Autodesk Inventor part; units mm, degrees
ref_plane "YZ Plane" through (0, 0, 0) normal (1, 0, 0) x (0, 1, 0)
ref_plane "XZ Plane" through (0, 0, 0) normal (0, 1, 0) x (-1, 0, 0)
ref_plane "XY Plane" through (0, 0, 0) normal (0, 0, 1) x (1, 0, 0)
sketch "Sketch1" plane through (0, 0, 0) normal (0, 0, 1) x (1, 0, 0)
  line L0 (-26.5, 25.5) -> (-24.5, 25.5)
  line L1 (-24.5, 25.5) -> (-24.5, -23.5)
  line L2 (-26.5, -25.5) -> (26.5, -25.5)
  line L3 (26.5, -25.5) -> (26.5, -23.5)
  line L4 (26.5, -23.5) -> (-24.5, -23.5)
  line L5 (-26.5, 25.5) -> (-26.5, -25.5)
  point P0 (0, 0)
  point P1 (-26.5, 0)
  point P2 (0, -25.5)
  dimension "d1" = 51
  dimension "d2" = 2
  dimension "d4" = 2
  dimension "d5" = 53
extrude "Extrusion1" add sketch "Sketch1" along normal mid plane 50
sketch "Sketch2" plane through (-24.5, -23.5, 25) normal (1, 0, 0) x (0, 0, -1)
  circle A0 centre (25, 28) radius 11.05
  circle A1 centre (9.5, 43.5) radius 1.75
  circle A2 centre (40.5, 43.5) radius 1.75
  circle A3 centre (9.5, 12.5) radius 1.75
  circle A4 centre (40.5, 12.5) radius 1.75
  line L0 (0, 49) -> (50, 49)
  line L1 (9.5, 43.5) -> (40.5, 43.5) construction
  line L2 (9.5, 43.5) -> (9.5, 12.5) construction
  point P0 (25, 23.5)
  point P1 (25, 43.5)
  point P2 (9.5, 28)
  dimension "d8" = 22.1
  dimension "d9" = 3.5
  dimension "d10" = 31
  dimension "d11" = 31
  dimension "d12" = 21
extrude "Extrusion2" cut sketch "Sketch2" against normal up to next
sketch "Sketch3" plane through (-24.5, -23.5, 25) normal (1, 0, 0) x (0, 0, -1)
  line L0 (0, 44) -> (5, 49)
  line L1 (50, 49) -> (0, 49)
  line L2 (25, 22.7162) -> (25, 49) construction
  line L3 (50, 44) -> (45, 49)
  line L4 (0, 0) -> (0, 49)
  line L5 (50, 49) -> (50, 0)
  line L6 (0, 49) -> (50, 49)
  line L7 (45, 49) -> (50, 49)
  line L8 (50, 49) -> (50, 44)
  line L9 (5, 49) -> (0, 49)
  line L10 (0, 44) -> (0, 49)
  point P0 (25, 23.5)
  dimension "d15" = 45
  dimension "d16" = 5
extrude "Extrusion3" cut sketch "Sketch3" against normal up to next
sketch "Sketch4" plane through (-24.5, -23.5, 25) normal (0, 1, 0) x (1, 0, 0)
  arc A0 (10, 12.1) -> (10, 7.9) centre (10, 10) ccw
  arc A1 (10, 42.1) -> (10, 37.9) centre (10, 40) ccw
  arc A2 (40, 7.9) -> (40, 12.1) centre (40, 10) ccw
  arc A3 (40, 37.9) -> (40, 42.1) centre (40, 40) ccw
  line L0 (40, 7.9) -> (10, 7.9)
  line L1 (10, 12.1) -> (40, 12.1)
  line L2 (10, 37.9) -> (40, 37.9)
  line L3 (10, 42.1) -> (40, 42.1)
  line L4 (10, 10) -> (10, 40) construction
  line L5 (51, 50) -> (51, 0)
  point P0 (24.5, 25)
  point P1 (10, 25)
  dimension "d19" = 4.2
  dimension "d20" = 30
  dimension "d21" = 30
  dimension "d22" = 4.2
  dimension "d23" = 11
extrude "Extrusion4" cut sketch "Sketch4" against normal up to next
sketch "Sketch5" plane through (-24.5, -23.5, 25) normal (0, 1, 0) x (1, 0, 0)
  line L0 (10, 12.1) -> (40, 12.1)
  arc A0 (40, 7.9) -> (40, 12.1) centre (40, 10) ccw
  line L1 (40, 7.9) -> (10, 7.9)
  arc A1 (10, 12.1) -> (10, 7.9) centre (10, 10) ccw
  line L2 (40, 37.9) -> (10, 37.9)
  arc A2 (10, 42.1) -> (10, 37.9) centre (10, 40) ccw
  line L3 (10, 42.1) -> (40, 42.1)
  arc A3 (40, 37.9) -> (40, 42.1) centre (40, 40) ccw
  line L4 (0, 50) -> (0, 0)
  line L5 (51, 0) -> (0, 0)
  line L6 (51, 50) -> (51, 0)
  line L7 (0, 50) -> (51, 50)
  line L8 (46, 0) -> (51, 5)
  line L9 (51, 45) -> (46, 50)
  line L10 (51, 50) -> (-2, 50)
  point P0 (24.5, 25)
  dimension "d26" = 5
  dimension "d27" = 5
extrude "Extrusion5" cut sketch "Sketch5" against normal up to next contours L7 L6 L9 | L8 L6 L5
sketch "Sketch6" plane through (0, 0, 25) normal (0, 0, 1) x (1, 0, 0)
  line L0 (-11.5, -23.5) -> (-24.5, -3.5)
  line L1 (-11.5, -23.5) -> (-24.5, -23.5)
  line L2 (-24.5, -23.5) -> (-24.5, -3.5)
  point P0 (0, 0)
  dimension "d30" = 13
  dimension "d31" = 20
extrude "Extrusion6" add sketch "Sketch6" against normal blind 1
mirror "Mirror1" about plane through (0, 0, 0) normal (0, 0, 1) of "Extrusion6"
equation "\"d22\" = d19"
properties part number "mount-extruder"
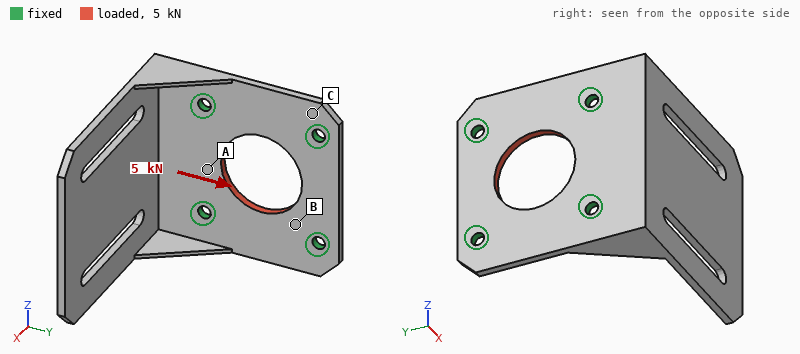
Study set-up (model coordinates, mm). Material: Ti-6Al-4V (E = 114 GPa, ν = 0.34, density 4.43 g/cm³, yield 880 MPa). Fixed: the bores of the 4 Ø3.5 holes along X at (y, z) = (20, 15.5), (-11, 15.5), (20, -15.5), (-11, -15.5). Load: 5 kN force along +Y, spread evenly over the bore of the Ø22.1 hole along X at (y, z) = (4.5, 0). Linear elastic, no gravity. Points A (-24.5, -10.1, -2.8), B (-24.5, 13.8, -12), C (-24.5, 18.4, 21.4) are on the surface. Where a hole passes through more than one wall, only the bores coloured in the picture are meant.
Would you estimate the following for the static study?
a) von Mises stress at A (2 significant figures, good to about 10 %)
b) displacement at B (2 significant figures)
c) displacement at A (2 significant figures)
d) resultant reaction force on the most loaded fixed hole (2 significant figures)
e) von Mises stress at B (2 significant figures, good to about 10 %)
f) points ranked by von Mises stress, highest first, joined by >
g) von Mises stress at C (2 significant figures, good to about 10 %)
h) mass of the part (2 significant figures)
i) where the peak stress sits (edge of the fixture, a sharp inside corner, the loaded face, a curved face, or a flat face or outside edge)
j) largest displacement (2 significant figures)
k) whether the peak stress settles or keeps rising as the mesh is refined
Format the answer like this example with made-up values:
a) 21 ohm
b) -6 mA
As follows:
a) 29 MPa
b) 4.6 µm
c) 6.7 µm
d) 1.3 kN
e) 53 MPa
f) B > A > C
g) 12 MPa
h) 40 g
i) edge of the fixture
j) 14 µm
k) keeps rising
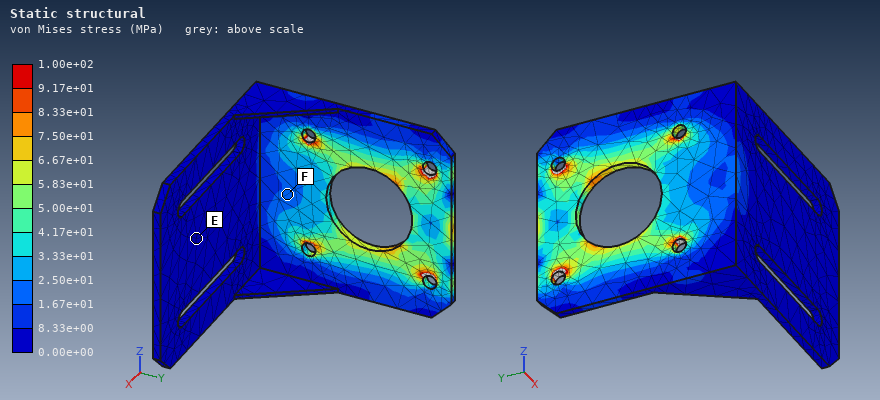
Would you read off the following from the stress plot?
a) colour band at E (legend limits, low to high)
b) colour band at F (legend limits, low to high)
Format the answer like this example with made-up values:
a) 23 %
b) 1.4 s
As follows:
a) 0.00e+00 to 8.33e+00 MPa
b) 1.67e+01 to 2.50e+01 MPa
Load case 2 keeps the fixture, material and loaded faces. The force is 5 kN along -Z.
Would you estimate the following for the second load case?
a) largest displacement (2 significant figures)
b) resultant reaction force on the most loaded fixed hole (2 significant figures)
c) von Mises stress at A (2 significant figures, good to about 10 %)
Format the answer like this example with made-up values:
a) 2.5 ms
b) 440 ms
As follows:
a) 11 µm
b) 1.3 kN
c) 42 MPa
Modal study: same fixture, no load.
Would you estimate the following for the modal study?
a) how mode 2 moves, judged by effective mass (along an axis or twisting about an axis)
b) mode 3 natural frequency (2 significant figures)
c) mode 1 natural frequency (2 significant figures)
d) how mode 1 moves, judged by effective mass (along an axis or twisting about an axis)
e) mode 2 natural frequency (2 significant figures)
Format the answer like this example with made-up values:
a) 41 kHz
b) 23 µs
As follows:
a) along Z
b) 2200 Hz
c) 590 Hz
d) along Y
e) 1400 Hz
